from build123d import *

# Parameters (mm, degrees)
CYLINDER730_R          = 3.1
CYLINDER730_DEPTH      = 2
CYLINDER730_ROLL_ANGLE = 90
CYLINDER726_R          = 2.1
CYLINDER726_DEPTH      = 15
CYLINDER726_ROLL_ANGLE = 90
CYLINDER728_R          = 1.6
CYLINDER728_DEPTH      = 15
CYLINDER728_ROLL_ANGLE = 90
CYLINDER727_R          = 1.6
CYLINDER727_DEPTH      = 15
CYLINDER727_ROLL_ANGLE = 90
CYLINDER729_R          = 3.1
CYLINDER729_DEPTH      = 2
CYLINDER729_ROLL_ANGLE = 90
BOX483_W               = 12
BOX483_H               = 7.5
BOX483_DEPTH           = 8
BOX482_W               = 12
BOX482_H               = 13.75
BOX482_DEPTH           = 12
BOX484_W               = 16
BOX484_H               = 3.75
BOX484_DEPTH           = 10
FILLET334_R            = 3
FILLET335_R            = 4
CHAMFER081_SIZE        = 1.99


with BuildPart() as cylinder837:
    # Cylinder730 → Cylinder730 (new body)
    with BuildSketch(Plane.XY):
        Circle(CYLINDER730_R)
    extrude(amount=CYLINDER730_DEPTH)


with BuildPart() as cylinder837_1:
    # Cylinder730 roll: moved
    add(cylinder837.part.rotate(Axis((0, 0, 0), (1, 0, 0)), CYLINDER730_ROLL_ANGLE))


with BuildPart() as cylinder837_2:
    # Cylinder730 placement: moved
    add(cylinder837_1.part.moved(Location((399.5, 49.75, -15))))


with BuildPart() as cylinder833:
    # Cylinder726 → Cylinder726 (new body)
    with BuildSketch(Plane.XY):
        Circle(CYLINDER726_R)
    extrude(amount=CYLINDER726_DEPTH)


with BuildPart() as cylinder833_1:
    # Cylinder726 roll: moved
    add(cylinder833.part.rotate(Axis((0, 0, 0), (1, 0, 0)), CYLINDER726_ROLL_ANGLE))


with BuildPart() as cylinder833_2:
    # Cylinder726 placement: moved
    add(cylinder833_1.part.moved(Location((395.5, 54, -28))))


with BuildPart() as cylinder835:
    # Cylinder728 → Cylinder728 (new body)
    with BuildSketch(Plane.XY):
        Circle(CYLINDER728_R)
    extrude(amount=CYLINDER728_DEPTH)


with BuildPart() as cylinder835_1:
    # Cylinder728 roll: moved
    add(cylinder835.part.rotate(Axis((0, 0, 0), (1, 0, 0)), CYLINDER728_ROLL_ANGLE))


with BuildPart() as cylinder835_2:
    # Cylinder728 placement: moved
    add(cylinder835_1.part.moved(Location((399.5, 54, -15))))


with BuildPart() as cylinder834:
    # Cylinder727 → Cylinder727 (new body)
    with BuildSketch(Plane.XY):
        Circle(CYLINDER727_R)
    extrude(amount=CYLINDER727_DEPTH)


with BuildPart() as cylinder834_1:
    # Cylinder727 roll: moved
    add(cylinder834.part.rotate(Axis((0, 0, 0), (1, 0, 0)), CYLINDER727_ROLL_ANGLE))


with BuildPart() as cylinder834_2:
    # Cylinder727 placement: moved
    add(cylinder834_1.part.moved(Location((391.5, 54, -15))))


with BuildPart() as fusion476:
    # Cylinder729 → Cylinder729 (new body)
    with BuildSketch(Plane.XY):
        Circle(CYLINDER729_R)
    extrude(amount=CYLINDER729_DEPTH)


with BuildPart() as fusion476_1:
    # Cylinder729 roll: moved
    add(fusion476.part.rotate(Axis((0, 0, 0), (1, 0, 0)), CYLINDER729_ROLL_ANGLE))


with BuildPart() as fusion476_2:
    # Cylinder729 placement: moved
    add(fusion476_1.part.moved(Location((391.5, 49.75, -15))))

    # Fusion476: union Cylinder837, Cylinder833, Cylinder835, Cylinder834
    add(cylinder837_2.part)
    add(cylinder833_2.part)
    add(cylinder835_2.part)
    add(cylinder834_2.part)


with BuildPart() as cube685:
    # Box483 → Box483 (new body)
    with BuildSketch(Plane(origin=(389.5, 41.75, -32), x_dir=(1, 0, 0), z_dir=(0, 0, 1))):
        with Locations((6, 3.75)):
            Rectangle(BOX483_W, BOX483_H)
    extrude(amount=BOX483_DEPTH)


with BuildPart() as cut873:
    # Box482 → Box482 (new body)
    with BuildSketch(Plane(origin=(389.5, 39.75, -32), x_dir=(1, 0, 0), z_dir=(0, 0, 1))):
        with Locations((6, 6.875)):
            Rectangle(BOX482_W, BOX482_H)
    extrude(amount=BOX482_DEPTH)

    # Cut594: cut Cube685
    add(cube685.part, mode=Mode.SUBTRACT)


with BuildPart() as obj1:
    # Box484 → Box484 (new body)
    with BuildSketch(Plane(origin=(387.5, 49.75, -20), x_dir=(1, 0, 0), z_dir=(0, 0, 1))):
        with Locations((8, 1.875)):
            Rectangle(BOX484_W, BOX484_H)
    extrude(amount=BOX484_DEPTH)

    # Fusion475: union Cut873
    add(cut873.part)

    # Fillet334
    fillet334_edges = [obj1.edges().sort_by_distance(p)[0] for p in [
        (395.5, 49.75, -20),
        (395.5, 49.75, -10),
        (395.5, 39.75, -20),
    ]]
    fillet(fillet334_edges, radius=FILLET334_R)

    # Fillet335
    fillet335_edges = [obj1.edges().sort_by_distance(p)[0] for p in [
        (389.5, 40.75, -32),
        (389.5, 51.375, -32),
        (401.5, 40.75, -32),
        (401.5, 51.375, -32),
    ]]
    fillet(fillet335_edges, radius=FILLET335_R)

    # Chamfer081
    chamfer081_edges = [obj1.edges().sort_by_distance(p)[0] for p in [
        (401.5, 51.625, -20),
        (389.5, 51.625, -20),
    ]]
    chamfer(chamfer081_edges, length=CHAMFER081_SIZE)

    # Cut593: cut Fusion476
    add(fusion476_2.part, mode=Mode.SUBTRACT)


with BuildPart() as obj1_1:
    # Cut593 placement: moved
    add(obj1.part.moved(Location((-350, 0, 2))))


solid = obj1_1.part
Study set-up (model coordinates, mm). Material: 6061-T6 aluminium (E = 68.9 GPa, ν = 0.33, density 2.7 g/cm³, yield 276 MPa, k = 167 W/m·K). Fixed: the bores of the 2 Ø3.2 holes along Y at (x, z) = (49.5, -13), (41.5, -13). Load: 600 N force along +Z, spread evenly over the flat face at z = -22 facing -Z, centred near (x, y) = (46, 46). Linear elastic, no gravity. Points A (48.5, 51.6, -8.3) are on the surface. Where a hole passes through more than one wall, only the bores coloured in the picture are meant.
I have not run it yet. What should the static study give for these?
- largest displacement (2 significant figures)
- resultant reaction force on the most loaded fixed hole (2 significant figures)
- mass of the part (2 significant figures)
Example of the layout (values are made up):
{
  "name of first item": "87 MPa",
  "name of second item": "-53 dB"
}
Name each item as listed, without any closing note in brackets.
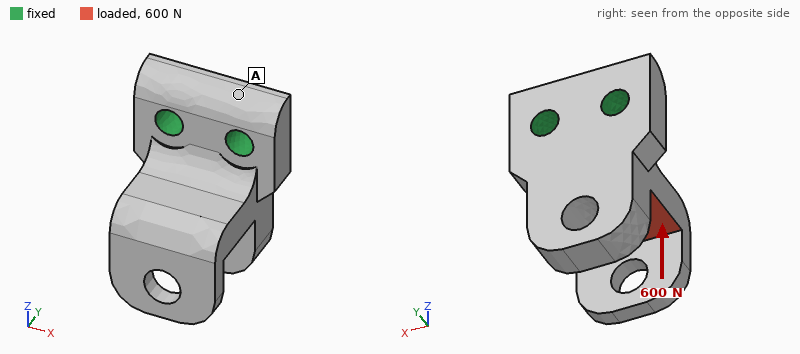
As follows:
{
  "largest displacement": "79 µm",
  "resultant reaction force on the most loaded fixed hole": "310 N",
  "mass of the part": "4.5 g"
}
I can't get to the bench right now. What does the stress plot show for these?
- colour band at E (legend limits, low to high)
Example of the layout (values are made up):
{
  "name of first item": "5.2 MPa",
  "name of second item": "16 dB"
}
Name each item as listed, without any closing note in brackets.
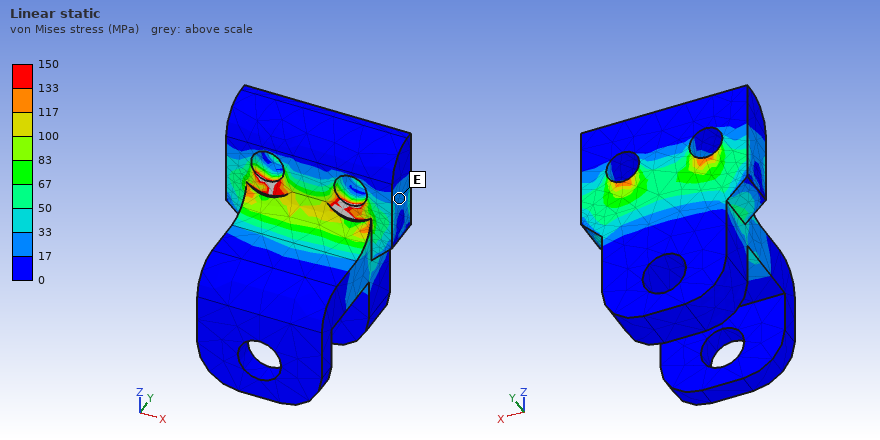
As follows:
{
  "colour band at E": "17 to 33 MPa"
}
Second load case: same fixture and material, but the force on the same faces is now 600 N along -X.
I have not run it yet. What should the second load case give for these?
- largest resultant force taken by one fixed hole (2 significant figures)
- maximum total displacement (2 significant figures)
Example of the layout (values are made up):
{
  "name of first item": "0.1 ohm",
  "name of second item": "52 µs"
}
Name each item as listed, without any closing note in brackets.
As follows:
{
  "largest resultant force taken by one fixed hole": "670 N",
  "maximum total displacement": "22 µm"
}
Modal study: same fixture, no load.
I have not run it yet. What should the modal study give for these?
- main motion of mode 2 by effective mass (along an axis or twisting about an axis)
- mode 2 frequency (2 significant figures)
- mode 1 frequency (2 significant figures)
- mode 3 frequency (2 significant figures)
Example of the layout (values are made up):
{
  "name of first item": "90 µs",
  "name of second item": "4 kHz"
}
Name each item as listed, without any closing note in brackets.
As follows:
{
  "main motion of mode 2 by effective mass": "along X",
  "mode 2 frequency": "20 kHz",
  "mode 1 frequency": "8900 Hz",
  "mode 3 frequency": "21 kHz"
}
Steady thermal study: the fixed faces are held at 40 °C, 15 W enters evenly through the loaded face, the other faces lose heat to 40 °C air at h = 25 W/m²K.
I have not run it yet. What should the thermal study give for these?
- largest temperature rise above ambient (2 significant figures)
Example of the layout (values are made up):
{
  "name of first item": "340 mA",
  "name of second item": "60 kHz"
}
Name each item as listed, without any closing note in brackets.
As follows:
{
  "largest temperature rise above ambient": "17 K"
}
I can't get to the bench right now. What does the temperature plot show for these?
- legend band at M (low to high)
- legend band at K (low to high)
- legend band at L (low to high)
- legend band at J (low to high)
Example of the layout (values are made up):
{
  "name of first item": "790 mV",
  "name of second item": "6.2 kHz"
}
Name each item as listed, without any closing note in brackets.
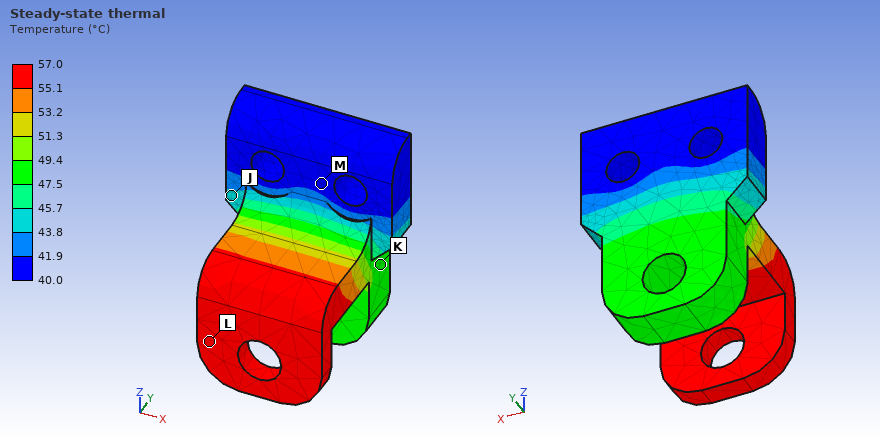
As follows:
{
  "legend band at M": "40.0 to 41.9 °C",
  "legend band at K": "47.5 to 49.4 °C",
  "legend band at L": "55.1 to 57.0 °C",
  "legend band at J": "43.8 to 45.7 °C"
}
